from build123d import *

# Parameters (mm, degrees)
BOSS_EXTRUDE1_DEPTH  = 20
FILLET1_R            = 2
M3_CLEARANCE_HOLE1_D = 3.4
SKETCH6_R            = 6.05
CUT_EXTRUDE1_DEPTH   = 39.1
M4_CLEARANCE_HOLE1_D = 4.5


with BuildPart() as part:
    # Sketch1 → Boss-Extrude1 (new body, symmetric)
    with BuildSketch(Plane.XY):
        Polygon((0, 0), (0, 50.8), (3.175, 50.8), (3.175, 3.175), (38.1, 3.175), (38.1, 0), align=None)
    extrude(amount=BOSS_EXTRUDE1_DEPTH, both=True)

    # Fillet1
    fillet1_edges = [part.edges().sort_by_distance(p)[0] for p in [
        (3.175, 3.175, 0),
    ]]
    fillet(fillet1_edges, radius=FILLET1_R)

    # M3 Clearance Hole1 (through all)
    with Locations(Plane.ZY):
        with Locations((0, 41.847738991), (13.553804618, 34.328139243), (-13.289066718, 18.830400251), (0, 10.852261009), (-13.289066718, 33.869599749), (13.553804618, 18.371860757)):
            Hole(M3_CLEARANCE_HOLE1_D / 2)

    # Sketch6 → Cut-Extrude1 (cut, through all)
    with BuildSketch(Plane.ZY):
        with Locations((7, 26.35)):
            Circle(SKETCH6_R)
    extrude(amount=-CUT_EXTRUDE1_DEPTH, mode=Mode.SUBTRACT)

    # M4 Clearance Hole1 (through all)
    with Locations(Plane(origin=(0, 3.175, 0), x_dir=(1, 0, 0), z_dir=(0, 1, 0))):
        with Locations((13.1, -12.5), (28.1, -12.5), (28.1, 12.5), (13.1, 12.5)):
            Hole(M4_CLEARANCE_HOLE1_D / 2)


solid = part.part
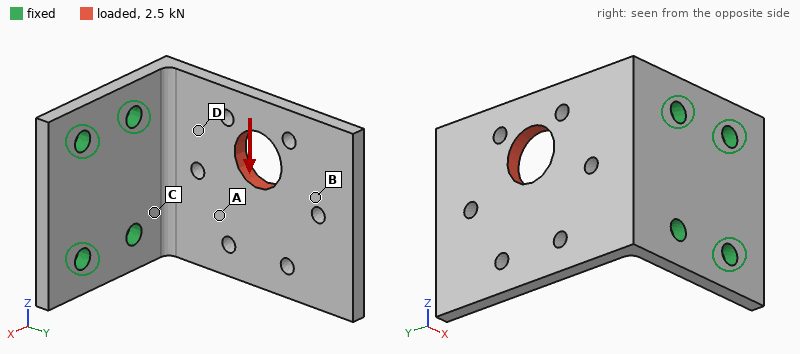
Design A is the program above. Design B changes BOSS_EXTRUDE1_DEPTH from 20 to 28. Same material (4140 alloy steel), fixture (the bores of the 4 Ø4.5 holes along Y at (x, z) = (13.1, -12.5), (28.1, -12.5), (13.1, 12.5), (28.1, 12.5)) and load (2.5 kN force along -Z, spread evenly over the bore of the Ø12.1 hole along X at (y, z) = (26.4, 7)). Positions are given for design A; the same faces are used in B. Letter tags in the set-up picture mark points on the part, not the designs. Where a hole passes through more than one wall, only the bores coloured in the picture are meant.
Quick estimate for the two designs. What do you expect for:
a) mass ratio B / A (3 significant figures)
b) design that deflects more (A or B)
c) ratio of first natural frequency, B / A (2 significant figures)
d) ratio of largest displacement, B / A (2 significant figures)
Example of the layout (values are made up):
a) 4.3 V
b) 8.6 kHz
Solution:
a) 1.43
b) A
c) 0.99
d) 0.85
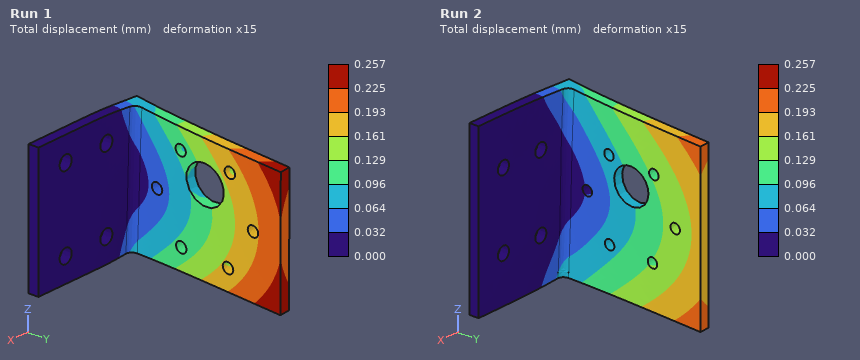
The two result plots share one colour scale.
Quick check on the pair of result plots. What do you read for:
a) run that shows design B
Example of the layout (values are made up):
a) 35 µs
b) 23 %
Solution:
a) Run 2
